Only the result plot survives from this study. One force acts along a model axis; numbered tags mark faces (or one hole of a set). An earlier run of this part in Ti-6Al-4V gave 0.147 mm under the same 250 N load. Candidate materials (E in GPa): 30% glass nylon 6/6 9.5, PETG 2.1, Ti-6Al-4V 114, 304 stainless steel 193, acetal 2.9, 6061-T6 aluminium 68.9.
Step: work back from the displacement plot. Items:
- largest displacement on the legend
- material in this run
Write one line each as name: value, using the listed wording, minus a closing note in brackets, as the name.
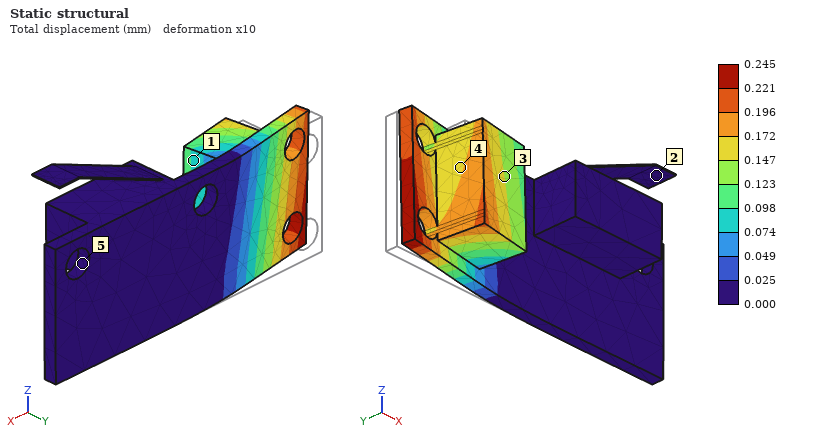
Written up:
largest displacement on the legend: 0.245 mm
material in this run: 6061-T6 aluminium
